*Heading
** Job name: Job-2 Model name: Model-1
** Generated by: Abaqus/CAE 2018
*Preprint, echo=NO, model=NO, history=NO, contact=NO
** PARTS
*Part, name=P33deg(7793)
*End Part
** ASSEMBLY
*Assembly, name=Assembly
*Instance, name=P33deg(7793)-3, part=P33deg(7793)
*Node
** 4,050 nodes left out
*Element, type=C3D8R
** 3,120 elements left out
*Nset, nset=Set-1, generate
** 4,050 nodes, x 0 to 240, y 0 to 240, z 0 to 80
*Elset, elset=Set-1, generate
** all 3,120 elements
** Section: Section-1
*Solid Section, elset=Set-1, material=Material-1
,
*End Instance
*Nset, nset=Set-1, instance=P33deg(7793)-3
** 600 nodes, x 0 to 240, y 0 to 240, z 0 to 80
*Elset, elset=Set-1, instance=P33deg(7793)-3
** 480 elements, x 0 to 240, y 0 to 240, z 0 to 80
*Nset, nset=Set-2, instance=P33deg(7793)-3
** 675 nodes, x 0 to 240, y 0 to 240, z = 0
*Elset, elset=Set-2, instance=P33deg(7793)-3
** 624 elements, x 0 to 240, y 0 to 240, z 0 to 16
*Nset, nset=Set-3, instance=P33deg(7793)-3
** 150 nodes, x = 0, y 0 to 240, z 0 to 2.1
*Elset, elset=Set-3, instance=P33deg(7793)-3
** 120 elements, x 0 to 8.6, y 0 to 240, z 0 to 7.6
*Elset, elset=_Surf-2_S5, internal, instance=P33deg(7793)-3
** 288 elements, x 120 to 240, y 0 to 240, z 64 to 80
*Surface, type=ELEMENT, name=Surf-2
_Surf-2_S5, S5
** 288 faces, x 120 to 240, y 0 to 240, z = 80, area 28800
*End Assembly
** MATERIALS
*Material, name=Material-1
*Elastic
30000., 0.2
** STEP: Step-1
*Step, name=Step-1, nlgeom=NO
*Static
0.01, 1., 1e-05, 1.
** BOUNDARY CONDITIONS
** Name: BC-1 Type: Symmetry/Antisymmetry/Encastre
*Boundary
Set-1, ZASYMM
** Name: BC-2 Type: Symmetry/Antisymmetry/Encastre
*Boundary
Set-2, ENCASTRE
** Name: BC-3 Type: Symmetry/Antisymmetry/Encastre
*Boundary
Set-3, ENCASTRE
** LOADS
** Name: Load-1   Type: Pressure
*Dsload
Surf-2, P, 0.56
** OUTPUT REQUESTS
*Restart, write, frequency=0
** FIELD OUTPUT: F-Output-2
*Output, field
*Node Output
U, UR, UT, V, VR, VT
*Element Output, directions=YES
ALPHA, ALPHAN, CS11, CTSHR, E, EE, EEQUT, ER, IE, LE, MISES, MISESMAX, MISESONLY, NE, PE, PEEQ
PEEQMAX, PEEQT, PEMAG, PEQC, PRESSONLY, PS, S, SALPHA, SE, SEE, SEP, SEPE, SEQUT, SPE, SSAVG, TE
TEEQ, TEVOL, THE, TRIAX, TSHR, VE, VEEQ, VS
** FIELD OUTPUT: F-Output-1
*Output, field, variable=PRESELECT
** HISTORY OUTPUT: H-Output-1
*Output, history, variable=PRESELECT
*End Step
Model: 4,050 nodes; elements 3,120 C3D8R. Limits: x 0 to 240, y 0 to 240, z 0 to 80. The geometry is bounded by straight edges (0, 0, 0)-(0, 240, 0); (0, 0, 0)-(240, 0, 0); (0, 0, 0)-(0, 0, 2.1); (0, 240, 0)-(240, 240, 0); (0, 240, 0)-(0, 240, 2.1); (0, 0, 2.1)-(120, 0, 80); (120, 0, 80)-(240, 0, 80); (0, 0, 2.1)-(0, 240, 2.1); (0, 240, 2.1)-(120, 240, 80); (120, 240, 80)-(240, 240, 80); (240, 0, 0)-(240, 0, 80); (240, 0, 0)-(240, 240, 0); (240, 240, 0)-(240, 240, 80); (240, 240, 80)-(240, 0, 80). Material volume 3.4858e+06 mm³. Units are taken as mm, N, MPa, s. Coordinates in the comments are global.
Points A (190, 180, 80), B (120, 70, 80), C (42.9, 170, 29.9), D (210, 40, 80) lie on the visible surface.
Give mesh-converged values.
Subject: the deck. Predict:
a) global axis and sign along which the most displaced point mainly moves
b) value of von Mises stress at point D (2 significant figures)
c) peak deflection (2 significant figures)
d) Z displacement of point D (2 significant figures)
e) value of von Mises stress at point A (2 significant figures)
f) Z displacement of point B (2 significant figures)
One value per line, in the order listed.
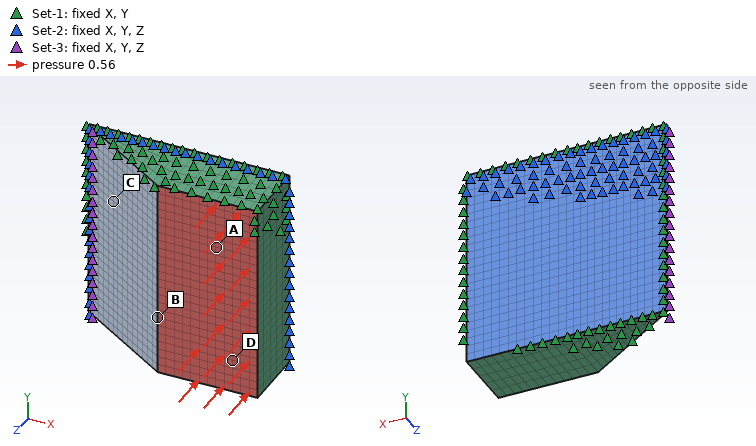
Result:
-Z
0.41 MPa
0.0014 mm
-0.0013 mm
0.39 MPa
-6.8e-04 mm
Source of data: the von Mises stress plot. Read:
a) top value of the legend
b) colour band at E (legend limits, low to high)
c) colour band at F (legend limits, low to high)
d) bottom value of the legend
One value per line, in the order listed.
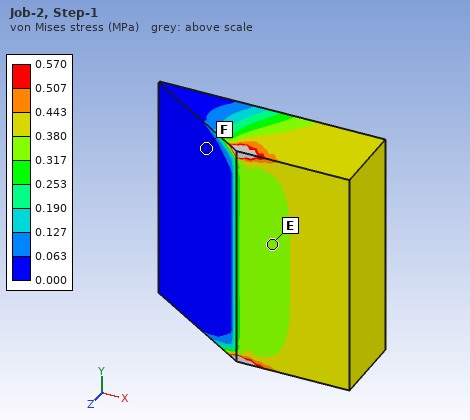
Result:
0.570 MPa
0.317 to 0.380 MPa
0.000 to 0.063 MPa
0.000 MPa
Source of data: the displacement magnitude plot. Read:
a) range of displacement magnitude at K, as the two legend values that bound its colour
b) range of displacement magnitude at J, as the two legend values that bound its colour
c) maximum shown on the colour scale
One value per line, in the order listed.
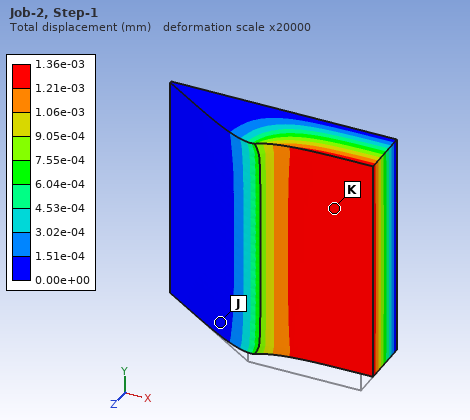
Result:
1.21e-03 to 1.36e-03 mm
0.00e+00 to 1.51e-04 mm
1.36e-03 mm
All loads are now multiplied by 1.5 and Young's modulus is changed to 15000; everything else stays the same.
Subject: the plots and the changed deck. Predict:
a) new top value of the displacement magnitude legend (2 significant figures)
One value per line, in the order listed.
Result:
0.0041 mm
